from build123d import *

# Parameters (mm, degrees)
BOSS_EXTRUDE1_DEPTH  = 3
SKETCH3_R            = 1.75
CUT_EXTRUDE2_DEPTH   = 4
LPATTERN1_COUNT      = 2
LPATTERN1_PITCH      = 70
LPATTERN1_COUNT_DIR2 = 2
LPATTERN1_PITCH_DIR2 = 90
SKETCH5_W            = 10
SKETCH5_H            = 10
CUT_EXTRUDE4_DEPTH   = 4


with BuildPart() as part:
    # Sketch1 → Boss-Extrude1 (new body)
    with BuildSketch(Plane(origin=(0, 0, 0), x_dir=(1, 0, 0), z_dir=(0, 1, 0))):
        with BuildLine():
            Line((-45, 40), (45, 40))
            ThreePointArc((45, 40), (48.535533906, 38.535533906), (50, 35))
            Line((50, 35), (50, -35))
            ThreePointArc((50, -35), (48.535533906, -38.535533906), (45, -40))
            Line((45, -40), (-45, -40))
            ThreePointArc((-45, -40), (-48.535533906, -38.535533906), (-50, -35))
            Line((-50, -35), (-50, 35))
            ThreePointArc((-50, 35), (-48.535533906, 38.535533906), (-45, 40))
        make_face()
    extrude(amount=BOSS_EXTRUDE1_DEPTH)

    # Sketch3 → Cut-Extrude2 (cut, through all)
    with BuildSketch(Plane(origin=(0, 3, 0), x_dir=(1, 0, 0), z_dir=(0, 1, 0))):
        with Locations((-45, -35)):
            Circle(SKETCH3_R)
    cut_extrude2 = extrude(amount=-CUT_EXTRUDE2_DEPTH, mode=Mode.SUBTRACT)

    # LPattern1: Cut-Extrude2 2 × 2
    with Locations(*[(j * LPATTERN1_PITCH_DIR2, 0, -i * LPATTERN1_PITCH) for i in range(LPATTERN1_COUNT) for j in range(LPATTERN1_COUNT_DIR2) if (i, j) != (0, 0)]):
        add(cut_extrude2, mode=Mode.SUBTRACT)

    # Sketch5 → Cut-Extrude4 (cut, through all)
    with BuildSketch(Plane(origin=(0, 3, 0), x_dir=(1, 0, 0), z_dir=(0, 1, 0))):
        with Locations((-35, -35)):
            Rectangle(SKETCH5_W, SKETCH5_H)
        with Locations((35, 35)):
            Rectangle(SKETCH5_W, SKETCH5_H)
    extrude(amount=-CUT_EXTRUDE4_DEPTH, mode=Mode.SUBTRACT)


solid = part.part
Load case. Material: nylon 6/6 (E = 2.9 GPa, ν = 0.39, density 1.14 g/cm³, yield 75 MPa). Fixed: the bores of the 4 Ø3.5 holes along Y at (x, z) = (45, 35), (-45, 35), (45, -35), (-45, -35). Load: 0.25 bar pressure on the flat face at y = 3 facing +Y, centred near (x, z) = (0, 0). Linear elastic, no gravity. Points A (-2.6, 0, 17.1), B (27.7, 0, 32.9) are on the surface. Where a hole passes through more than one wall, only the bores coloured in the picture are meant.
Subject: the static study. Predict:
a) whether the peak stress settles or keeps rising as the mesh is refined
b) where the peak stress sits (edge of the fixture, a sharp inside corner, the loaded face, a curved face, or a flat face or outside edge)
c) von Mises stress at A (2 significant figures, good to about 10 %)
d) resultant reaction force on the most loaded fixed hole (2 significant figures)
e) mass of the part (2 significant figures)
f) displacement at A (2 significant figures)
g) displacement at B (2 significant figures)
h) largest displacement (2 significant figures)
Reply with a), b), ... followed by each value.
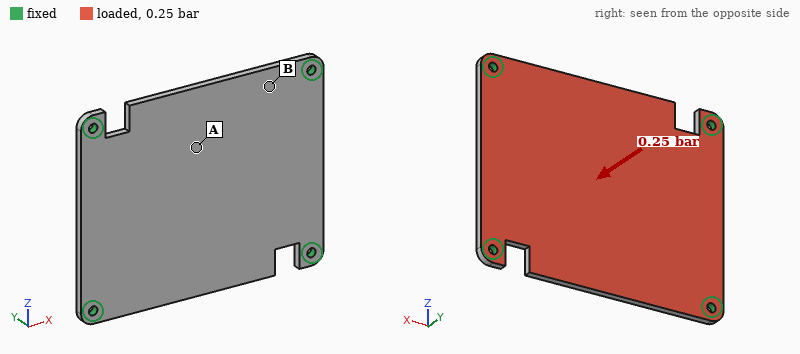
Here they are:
a) keeps rising
b) edge of the fixture
c) 7.4 MPa
d) 53 N
e) 26 g
f) 1.3 mm
g) 0.51 mm
h) 1.4 mm
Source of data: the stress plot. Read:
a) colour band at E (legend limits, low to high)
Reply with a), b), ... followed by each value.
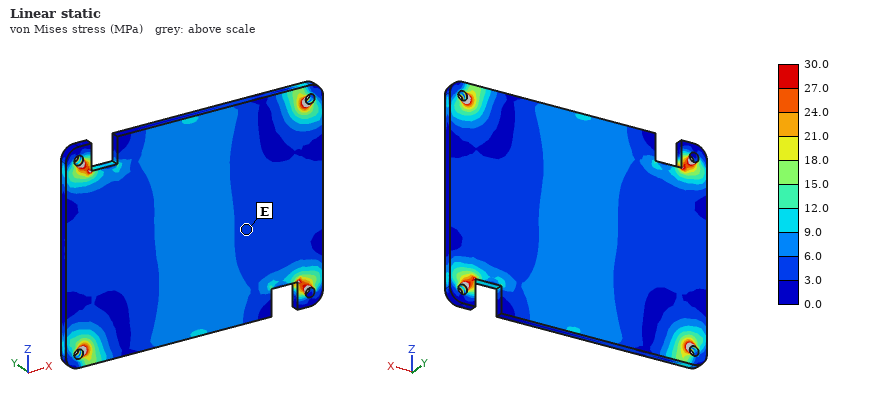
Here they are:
a) 3.0 to 6.0 MPa
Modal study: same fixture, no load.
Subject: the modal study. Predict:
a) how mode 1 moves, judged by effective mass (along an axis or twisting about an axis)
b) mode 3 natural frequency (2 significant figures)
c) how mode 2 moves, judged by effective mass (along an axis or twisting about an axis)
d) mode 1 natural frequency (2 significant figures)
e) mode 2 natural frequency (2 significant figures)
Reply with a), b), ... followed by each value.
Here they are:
a) along Y
b) 940 Hz
c) twisting about X
d) 420 Hz
e) 630 Hz
